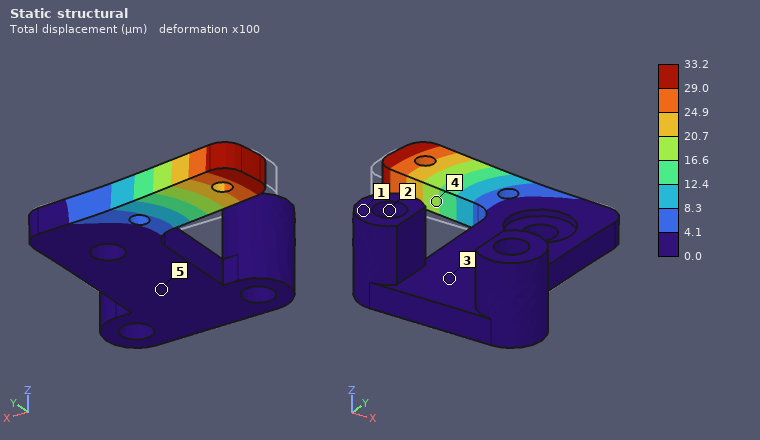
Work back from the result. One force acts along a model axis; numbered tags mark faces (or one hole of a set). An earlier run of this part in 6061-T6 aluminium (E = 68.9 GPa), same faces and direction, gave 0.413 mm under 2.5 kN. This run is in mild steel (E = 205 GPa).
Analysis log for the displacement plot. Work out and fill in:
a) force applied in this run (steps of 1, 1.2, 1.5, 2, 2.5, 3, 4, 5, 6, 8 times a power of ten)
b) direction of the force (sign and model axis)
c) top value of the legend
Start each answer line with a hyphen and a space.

- 600 N
- +Y
- 33.2 µm
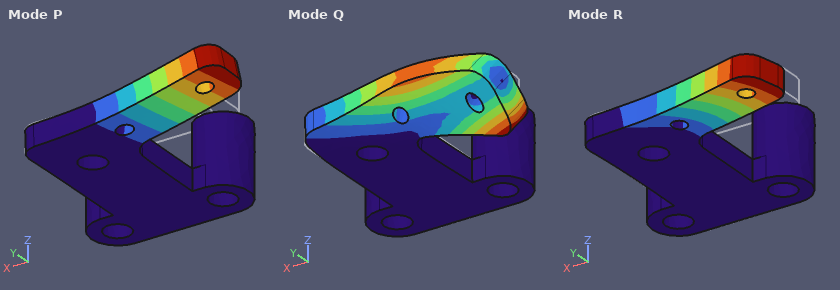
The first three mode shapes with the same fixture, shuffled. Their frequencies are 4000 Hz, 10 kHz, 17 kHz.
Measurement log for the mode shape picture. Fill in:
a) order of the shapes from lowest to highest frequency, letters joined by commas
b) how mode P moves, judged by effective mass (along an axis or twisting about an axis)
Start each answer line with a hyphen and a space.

- P, R, Q
- along Z
